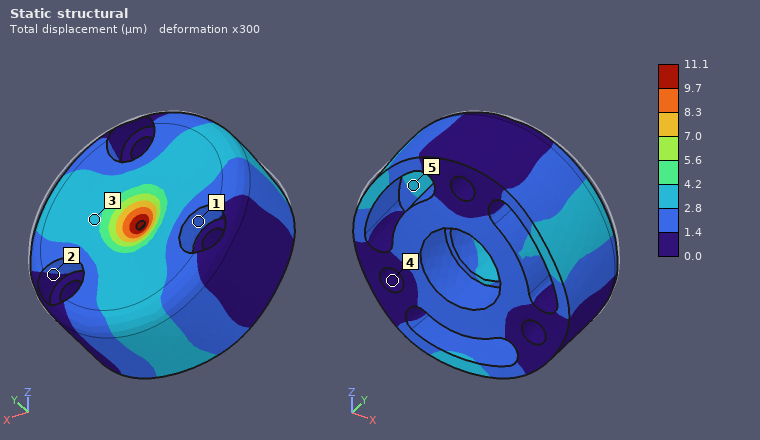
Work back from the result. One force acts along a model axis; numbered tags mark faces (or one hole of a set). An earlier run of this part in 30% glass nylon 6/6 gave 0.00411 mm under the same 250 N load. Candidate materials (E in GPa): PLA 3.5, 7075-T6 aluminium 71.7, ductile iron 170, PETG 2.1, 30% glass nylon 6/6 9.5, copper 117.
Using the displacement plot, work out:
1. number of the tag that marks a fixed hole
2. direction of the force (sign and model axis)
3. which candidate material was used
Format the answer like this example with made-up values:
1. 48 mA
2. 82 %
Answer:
1. 4
2. -Y
3. PLA
